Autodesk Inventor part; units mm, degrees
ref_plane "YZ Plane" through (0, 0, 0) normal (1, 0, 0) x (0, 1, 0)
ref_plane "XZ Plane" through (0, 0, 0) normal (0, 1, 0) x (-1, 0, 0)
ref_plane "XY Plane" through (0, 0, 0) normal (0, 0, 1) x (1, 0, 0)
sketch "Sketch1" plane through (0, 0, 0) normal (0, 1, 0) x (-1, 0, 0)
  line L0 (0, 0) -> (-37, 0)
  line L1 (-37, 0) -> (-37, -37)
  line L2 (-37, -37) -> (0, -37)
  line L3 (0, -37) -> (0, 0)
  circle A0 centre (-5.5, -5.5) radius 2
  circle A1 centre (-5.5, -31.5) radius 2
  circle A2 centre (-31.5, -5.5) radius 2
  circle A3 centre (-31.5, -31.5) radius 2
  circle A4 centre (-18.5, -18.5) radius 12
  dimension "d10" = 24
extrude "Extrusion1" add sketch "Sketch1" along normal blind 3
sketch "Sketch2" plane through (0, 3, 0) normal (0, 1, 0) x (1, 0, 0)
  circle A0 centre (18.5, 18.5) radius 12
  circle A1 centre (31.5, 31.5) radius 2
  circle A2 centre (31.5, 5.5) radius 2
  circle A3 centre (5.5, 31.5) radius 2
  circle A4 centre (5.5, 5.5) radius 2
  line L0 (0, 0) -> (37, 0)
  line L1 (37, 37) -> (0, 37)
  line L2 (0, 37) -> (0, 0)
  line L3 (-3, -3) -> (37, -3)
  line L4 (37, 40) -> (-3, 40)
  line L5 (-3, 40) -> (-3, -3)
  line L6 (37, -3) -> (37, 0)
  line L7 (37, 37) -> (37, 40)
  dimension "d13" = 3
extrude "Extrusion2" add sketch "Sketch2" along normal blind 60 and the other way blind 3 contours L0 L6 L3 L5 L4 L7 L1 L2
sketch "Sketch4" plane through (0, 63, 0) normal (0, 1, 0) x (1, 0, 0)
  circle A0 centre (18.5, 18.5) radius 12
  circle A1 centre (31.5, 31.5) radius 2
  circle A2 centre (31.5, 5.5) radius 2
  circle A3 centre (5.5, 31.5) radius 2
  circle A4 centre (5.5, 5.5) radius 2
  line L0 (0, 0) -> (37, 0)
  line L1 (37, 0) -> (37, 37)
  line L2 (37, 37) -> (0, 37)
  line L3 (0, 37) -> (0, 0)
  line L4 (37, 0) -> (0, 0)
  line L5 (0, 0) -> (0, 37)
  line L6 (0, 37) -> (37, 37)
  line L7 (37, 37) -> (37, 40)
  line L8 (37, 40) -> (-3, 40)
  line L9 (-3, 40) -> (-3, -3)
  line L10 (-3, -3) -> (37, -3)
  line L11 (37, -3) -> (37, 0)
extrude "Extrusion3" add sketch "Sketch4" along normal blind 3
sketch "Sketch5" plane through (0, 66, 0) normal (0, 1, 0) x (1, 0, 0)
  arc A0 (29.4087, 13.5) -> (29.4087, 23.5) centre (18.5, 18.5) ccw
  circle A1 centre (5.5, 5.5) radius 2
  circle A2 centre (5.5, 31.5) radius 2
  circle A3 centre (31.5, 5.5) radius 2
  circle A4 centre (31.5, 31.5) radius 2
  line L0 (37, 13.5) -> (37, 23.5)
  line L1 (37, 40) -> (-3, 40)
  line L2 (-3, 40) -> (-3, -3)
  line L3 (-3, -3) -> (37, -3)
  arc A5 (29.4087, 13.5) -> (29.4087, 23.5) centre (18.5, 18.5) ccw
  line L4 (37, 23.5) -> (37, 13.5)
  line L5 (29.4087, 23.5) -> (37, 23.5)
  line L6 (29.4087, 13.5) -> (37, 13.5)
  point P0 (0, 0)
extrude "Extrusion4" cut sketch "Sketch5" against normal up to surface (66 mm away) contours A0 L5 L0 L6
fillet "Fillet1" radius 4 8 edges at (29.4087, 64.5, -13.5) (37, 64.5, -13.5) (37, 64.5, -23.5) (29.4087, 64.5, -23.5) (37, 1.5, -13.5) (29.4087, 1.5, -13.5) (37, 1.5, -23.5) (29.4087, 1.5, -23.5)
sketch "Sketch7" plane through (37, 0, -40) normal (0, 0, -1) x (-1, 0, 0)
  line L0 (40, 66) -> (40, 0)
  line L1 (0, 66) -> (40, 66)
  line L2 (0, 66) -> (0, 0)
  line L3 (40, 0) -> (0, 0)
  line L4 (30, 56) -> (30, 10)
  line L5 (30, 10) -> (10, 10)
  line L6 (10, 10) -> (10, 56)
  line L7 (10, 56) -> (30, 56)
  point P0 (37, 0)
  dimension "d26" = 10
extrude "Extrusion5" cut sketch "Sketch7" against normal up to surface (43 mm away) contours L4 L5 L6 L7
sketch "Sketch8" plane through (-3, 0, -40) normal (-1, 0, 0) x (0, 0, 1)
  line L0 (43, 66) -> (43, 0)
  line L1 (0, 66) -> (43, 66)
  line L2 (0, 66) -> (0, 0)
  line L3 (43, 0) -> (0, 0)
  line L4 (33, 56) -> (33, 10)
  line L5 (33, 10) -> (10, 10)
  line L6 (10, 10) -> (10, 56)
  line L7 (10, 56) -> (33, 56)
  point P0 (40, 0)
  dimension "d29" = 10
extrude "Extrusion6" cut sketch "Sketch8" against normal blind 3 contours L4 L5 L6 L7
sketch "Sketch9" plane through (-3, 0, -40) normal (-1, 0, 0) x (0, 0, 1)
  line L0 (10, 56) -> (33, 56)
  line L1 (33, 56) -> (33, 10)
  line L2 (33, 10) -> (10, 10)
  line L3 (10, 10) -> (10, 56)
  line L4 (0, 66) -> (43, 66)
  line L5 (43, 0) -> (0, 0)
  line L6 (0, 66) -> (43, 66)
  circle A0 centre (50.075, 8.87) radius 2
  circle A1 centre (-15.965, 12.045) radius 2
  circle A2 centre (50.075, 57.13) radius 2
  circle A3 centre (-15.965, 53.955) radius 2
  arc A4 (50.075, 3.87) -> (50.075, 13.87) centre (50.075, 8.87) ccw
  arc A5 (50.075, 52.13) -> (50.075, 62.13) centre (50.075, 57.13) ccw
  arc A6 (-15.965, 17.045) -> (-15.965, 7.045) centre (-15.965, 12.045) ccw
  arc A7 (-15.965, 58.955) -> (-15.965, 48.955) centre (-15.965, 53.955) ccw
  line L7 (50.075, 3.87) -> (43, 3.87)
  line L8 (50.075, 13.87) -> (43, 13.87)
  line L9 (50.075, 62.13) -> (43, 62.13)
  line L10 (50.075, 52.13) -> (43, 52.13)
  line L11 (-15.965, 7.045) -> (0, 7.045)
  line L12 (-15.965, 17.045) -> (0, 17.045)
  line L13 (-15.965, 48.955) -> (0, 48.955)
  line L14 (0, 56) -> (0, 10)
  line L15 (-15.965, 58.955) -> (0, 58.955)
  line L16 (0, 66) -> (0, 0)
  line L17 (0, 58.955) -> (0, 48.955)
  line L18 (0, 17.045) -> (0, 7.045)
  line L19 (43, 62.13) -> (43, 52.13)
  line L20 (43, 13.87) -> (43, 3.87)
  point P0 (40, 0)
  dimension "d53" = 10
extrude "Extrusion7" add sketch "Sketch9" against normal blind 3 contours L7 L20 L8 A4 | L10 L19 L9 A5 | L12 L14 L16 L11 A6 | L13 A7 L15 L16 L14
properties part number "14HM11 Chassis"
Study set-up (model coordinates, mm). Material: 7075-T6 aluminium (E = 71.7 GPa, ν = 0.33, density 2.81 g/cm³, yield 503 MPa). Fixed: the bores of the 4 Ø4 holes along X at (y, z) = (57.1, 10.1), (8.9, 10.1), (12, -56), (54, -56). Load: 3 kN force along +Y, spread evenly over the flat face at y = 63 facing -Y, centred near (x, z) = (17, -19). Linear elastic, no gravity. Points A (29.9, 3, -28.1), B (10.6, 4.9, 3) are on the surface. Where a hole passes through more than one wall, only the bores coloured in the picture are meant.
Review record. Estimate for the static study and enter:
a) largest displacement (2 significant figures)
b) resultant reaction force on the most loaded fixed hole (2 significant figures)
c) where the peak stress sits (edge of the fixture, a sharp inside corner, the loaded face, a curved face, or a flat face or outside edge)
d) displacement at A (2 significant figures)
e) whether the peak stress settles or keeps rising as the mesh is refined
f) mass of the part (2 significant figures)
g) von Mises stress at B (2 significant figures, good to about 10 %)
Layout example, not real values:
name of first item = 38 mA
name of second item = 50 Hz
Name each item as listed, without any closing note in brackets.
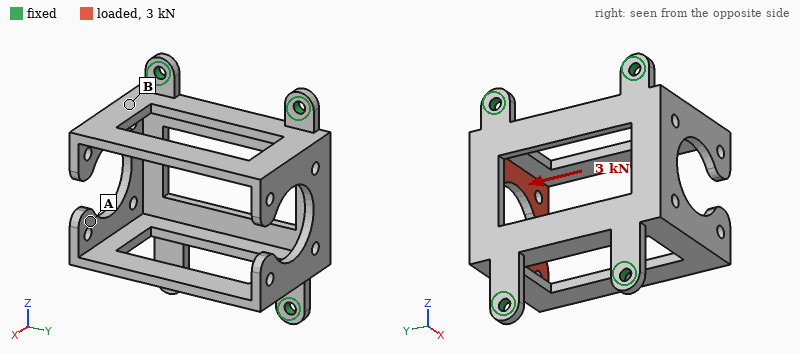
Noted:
largest displacement = 0.86 mm
resultant reaction force on the most loaded fixed hole = 1.1 kN
where the peak stress sits = edge of the fixture
displacement at A = 0.39 mm
whether the peak stress settles or keeps rising as the mesh is refined = keeps rising
mass of the part = 59 g
von Mises stress at B = 76 MPa
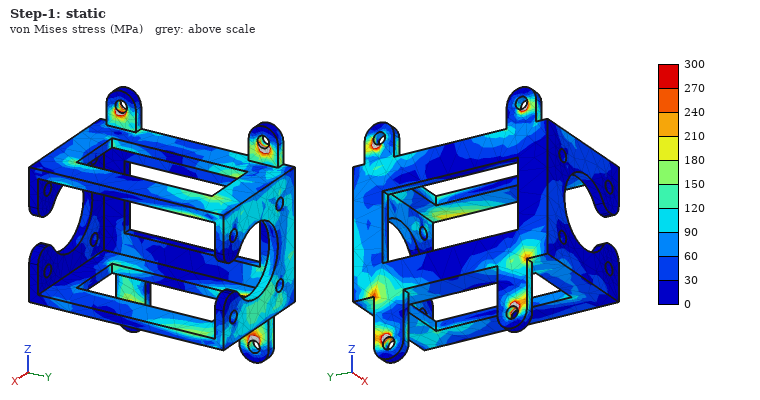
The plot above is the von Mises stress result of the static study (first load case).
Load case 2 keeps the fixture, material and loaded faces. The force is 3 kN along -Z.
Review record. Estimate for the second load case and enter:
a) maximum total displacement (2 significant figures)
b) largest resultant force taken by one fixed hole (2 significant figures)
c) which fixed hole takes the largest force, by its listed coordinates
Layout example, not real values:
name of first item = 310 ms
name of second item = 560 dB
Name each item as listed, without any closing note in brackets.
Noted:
maximum total displacement = 0.64 mm
largest resultant force taken by one fixed hole = 2.1 kN
which fixed hole takes the largest force, by its listed coordinates = (57.1, 10.1)
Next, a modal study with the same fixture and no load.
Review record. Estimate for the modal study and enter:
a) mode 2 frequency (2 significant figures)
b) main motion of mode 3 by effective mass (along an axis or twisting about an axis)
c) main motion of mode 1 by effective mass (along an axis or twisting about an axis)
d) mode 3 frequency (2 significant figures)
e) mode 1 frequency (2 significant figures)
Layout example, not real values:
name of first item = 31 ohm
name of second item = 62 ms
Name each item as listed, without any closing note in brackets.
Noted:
mode 2 frequency = 2100 Hz
main motion of mode 3 by effective mass = along Z
main motion of mode 1 by effective mass = along Y
mode 3 frequency = 2300 Hz
mode 1 frequency = 1900 Hz
